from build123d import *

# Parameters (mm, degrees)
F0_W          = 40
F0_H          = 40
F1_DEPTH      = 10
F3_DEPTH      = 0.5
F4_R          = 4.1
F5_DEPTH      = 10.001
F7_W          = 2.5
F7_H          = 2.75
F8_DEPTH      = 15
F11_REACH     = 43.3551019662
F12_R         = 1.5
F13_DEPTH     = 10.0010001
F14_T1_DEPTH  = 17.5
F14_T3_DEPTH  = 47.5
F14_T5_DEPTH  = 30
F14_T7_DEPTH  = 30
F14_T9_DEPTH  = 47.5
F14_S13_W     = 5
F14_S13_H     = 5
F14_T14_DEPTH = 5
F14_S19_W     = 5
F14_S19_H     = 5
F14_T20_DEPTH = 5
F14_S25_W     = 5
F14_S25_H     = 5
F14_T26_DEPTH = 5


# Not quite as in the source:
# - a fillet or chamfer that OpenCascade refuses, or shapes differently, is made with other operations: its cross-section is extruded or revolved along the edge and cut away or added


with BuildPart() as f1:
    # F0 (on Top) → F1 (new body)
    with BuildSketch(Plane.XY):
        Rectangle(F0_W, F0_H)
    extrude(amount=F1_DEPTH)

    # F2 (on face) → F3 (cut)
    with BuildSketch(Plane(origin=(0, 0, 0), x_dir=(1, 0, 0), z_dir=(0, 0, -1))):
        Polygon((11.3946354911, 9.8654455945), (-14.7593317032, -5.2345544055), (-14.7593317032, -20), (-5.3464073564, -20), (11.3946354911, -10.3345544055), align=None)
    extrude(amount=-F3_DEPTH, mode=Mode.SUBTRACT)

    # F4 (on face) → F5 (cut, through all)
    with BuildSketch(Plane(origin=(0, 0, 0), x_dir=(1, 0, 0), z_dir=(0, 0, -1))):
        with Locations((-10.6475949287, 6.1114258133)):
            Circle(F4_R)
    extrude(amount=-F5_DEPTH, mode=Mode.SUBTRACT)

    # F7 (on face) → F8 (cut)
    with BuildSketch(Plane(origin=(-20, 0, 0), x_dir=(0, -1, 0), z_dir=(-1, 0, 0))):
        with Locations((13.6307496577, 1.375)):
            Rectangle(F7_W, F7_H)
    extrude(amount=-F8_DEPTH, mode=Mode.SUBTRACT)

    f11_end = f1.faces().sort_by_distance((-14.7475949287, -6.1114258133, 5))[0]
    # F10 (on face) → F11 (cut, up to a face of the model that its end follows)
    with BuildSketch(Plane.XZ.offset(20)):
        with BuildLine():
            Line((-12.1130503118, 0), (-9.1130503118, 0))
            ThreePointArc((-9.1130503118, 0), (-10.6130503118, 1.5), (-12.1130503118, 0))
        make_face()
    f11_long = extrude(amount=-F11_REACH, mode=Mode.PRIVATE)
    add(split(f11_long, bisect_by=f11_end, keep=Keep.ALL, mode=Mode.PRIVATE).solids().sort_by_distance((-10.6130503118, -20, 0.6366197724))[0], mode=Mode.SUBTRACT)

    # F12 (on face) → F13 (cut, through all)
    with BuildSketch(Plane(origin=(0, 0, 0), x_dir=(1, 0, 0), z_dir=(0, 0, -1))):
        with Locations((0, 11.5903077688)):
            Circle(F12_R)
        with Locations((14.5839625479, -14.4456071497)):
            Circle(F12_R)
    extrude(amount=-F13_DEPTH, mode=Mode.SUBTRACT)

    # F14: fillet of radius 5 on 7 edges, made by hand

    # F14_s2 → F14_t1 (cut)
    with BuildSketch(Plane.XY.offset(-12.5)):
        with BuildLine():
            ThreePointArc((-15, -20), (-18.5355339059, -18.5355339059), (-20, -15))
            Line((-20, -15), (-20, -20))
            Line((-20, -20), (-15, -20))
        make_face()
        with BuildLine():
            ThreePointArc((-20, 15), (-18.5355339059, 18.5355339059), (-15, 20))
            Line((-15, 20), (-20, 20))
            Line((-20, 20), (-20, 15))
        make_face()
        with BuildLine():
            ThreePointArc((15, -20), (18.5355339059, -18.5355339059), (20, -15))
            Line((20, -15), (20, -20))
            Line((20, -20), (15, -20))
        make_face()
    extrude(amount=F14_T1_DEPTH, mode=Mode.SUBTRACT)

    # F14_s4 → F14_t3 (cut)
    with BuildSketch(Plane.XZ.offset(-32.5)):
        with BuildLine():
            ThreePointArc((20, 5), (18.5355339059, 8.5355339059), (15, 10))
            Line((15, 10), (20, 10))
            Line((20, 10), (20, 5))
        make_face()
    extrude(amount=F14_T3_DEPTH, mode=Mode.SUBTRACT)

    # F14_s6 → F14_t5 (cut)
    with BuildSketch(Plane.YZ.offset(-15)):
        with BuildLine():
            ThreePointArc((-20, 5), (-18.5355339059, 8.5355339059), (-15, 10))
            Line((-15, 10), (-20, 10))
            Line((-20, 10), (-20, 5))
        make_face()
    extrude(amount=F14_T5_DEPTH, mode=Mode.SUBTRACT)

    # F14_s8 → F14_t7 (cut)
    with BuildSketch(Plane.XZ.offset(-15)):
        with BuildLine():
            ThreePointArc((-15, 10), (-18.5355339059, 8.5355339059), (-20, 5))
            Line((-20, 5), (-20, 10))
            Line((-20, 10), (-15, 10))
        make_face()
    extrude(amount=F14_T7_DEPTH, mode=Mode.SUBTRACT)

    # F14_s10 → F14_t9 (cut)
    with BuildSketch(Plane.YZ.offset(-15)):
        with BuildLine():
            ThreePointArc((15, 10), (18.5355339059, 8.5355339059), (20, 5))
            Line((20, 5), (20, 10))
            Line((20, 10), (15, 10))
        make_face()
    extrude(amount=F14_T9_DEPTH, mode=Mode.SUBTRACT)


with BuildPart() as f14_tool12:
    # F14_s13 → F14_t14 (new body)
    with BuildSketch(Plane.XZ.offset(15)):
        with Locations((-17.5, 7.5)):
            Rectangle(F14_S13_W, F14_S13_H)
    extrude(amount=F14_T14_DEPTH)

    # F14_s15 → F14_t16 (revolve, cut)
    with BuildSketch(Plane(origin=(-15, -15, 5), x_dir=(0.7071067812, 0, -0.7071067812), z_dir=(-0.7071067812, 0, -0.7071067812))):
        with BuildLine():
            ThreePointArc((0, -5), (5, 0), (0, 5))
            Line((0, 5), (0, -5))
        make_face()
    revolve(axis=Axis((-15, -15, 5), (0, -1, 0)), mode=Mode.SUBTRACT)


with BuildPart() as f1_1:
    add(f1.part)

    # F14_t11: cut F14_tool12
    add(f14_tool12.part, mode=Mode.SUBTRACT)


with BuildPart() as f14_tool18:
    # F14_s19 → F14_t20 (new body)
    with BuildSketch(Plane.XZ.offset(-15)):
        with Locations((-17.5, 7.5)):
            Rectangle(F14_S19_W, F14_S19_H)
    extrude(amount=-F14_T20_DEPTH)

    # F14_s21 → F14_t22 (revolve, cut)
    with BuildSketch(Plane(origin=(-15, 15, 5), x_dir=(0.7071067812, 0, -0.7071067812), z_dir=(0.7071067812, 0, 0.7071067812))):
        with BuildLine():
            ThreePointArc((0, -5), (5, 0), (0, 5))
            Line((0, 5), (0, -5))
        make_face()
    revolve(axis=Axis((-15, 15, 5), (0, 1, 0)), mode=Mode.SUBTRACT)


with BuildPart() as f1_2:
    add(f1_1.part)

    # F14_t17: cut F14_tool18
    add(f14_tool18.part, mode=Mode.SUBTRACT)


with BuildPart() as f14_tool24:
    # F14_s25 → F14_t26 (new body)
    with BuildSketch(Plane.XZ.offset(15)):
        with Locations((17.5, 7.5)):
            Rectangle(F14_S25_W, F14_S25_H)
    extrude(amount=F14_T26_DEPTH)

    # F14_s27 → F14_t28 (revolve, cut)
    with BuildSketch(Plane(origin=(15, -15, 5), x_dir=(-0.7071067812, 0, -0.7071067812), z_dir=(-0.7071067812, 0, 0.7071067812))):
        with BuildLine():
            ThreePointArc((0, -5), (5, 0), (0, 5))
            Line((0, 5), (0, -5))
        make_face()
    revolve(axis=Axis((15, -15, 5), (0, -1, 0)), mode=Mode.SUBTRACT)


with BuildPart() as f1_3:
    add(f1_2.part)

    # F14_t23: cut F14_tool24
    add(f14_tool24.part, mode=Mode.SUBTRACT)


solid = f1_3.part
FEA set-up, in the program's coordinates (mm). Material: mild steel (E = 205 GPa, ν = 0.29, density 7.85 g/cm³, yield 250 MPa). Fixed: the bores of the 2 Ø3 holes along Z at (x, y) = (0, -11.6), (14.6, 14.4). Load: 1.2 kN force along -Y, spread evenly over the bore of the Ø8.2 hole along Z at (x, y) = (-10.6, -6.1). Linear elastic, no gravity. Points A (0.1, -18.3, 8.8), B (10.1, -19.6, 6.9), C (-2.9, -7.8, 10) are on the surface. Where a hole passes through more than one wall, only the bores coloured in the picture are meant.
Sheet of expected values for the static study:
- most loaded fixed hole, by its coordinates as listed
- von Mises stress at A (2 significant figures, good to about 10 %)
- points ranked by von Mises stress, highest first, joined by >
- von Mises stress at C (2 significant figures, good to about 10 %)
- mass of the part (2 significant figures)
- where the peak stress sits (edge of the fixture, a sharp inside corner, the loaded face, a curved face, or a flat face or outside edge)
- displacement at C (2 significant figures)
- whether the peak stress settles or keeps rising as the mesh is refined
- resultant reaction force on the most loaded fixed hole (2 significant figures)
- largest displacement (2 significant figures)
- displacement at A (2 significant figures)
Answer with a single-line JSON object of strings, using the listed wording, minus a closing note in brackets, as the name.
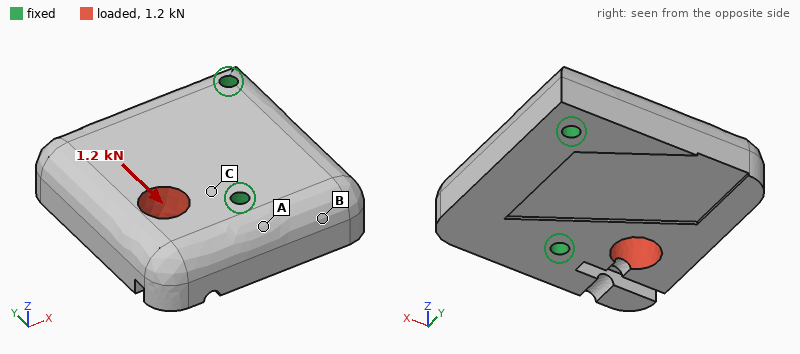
{"most loaded fixed hole, by its coordinates as listed": "(0, -11.6)", "von Mises stress at A": "8.1 MPa", "points ranked by von Mises stress, highest first, joined by >": "C > A > B", "von Mises stress at C": "14 MPa", "mass of the part": "110 g", "where the peak stress sits": "edge of the fixture", "displacement at C": "0.33 µm", "whether the peak stress settles or keeps rising as the mesh is refined": "keeps rising", "resultant reaction force on the most loaded fixed hole": "1.2 kN", "largest displacement": "1.7 µm", "displacement at A": "0.34 µm"}
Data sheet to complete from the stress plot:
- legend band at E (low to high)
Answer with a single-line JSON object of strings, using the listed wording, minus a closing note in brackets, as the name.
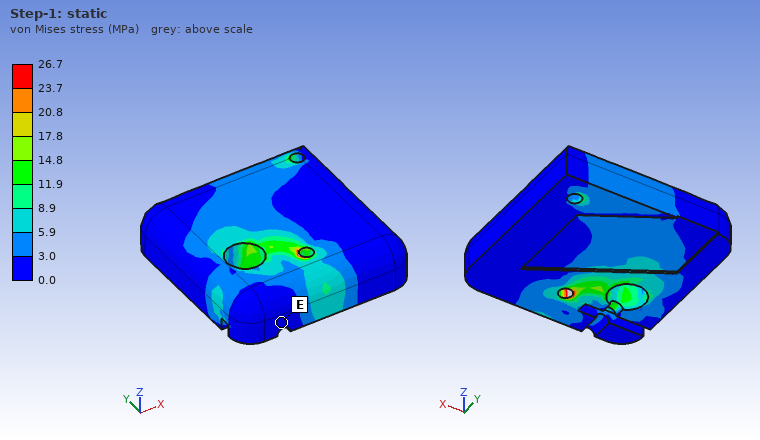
{"legend band at E": "0.0 to 3.0 MPa"}
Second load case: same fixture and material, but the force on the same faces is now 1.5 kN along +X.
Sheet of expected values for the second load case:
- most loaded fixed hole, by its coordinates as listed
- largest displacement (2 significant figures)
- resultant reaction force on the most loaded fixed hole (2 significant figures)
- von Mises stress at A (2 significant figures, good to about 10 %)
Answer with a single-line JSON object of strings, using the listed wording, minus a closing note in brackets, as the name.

{"most loaded fixed hole, by its coordinates as listed": "(0, -11.6)", "largest displacement": "1.2 µm", "resultant reaction force on the most loaded fixed hole": "1.1 kN", "von Mises stress at A": "3.5 MPa"}
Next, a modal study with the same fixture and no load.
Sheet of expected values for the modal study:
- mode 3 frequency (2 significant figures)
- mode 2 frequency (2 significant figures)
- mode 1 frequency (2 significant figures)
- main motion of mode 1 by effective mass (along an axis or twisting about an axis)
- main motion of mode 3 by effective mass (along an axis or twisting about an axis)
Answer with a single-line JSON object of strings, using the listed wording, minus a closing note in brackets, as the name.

{"mode 3 frequency": "21 kHz", "mode 2 frequency": "19 kHz", "mode 1 frequency": "8700 Hz", "main motion of mode 1 by effective mass": "along Z", "main motion of mode 3 by effective mass": "along Z"}
